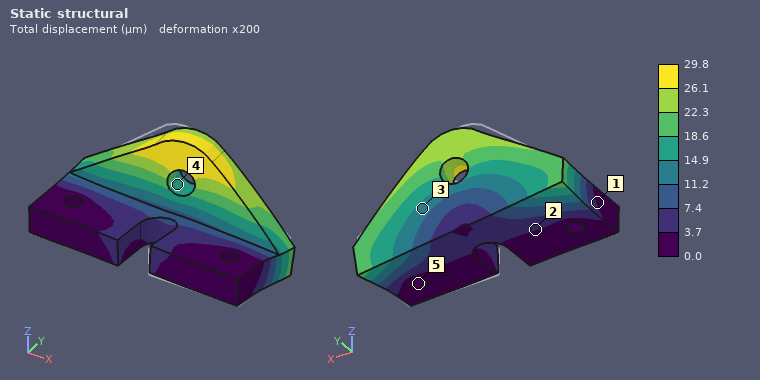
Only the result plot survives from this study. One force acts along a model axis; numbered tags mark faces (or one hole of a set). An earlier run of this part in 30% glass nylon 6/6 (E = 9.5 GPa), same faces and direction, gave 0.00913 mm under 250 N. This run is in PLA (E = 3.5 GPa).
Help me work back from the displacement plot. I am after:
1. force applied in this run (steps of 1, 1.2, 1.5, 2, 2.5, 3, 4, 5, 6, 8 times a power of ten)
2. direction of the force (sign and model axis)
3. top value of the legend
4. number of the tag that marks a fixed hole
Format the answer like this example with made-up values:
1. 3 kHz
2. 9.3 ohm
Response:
1. 300 N
2. +X
3. 29.8 µm
4. 5
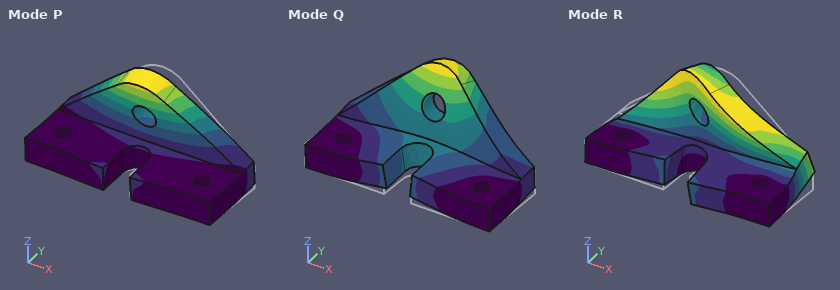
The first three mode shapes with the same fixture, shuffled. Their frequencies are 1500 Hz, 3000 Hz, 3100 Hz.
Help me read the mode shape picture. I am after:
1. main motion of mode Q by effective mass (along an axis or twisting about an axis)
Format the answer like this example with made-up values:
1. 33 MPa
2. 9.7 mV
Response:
1. along Z
